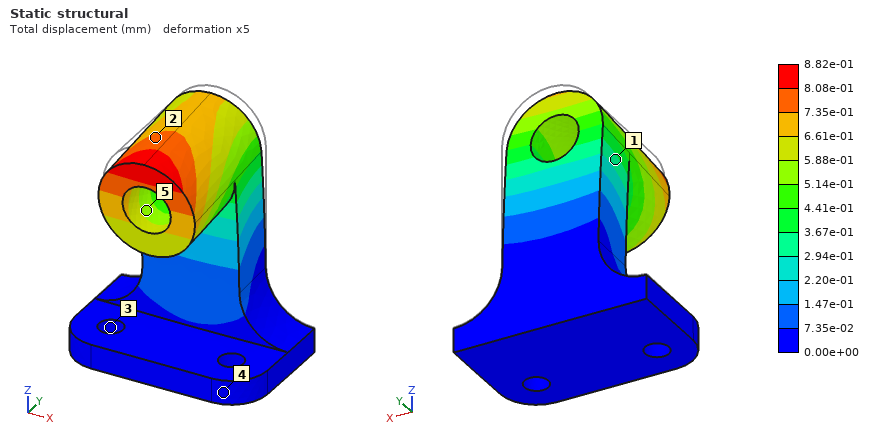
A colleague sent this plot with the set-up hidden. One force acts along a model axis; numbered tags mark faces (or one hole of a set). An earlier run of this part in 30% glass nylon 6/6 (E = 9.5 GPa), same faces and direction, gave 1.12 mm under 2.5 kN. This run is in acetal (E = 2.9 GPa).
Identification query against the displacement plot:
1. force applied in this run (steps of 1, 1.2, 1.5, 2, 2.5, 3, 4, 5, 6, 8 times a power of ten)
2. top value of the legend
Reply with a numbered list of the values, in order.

1. 600 N
2. 8.82e-01 mm
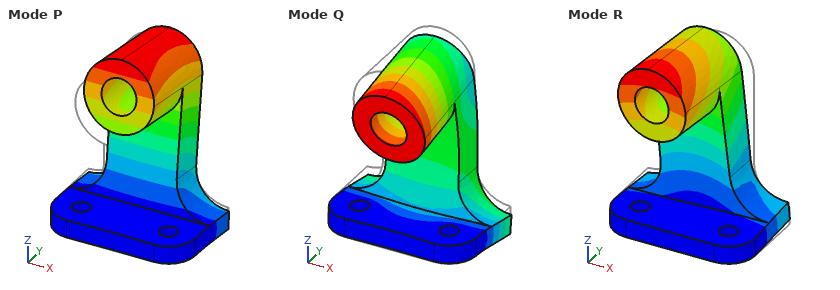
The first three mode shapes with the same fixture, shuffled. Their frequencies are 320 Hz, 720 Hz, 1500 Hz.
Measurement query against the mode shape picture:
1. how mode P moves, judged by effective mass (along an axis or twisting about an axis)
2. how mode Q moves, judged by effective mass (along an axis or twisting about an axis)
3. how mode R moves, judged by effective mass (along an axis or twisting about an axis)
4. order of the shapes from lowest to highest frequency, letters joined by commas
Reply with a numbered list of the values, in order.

1. along Y
2. along Z
3. along X
4. P, R, Q
